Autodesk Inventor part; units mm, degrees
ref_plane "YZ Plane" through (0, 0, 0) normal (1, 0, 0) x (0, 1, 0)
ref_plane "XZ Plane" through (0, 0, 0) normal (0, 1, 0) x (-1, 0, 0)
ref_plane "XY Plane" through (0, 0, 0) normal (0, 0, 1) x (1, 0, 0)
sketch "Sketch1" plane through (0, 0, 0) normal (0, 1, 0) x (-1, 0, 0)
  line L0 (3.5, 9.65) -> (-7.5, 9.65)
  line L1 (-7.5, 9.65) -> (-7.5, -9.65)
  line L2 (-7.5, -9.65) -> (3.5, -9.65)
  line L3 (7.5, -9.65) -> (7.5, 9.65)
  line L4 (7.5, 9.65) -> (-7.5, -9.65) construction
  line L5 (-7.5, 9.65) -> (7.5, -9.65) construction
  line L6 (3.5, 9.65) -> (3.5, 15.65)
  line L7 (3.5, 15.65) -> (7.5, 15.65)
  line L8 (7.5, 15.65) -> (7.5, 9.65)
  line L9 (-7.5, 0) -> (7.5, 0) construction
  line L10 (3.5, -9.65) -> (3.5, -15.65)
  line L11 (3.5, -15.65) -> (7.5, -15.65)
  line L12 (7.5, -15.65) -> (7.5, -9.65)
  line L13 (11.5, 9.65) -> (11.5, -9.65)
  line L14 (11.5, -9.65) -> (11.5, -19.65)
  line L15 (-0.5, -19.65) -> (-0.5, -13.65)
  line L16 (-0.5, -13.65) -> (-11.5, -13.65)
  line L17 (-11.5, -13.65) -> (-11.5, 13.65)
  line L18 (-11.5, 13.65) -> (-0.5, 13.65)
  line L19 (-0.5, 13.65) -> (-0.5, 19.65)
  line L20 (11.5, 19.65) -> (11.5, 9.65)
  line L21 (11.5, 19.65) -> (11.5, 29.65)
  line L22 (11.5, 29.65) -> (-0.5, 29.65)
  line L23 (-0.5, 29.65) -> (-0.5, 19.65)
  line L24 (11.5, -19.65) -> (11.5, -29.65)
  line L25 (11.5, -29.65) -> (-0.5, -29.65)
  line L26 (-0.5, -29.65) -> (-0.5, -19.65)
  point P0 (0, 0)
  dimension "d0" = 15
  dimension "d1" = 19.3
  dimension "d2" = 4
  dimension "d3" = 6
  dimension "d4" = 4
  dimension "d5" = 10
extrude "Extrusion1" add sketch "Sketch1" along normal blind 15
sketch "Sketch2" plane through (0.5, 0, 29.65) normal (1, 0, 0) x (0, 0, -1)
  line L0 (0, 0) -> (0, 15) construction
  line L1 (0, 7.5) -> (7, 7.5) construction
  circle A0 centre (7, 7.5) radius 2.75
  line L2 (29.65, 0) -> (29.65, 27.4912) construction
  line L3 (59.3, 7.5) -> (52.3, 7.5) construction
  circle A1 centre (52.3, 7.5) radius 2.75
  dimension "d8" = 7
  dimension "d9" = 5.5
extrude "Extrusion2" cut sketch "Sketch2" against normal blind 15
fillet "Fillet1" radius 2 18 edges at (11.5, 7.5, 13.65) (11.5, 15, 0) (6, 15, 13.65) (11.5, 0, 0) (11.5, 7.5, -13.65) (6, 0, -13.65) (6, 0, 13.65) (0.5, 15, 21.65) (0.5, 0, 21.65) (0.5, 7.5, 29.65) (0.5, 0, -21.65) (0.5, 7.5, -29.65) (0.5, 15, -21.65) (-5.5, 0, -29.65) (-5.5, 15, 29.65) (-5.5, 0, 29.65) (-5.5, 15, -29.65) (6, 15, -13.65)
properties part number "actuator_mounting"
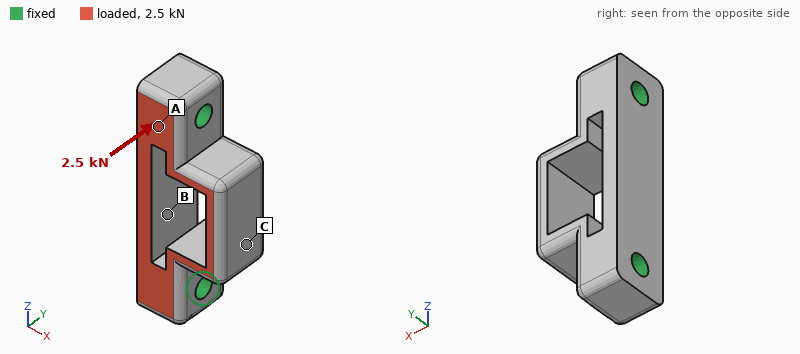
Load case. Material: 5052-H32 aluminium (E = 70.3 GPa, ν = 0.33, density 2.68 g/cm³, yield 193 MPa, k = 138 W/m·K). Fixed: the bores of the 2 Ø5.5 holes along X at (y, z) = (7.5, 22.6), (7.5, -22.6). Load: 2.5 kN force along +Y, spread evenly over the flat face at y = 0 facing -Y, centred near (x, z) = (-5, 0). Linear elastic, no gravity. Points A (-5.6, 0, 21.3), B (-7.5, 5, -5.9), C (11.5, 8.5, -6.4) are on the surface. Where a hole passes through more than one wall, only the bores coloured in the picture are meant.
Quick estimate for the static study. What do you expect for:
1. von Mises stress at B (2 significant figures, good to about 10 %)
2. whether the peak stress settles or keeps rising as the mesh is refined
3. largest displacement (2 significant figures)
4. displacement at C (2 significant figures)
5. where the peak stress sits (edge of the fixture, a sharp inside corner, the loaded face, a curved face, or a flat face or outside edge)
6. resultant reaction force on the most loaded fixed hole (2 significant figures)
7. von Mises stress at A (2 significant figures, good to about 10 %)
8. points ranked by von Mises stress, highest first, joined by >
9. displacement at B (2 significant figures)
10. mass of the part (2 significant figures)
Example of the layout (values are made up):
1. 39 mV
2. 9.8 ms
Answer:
1. 6.6 MPa
2. keeps rising
3. 14 µm
4. 13 µm
5. edge of the fixture
6. 1.3 kN
7. 14 MPa
8. A > B > C
9. 6.3 µm
10. 25 g
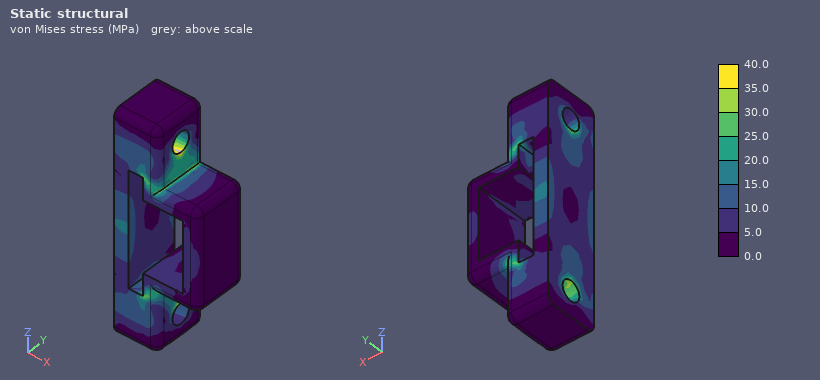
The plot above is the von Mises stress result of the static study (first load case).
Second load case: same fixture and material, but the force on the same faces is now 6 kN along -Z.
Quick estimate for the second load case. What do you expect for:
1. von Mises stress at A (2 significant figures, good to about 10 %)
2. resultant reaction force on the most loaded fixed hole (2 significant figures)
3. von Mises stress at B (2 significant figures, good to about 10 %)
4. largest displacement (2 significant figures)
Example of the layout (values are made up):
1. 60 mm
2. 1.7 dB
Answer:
1. 22 MPa
2. 3.1 kN
3. 17 MPa
4. 32 µm
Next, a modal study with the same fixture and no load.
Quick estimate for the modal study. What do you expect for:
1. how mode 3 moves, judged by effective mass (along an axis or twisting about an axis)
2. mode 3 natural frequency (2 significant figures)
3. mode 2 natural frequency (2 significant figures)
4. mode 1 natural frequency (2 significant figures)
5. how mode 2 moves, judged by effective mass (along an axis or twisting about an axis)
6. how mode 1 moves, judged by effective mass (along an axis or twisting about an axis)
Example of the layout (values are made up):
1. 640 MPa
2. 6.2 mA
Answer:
1. along X
2. 16 kHz
3. 14 kHz
4. 12 kHz
5. along Z
6. along Y
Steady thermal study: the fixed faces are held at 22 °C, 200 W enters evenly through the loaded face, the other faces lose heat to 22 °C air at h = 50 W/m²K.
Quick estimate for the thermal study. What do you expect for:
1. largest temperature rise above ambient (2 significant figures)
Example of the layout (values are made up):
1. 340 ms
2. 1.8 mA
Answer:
1. 58 K
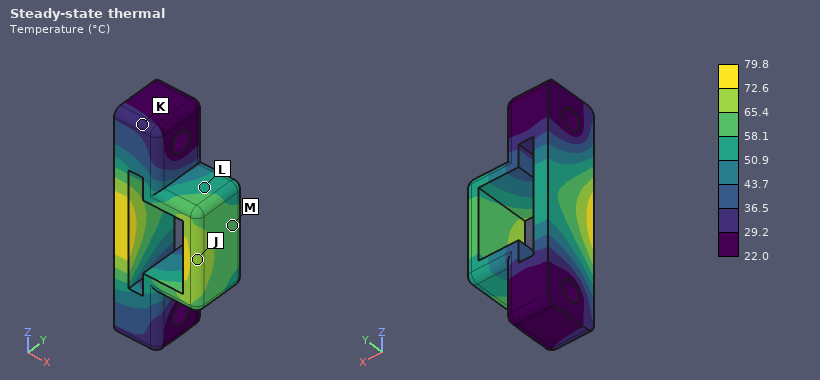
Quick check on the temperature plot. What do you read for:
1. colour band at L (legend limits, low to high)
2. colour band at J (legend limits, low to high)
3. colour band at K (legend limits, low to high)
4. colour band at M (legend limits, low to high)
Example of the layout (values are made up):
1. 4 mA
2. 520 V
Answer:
1. 50.9 to 58.1 °C
2. 65.4 to 72.6 °C
3. 29.2 to 36.5 °C
4. 58.1 to 65.4 °C
